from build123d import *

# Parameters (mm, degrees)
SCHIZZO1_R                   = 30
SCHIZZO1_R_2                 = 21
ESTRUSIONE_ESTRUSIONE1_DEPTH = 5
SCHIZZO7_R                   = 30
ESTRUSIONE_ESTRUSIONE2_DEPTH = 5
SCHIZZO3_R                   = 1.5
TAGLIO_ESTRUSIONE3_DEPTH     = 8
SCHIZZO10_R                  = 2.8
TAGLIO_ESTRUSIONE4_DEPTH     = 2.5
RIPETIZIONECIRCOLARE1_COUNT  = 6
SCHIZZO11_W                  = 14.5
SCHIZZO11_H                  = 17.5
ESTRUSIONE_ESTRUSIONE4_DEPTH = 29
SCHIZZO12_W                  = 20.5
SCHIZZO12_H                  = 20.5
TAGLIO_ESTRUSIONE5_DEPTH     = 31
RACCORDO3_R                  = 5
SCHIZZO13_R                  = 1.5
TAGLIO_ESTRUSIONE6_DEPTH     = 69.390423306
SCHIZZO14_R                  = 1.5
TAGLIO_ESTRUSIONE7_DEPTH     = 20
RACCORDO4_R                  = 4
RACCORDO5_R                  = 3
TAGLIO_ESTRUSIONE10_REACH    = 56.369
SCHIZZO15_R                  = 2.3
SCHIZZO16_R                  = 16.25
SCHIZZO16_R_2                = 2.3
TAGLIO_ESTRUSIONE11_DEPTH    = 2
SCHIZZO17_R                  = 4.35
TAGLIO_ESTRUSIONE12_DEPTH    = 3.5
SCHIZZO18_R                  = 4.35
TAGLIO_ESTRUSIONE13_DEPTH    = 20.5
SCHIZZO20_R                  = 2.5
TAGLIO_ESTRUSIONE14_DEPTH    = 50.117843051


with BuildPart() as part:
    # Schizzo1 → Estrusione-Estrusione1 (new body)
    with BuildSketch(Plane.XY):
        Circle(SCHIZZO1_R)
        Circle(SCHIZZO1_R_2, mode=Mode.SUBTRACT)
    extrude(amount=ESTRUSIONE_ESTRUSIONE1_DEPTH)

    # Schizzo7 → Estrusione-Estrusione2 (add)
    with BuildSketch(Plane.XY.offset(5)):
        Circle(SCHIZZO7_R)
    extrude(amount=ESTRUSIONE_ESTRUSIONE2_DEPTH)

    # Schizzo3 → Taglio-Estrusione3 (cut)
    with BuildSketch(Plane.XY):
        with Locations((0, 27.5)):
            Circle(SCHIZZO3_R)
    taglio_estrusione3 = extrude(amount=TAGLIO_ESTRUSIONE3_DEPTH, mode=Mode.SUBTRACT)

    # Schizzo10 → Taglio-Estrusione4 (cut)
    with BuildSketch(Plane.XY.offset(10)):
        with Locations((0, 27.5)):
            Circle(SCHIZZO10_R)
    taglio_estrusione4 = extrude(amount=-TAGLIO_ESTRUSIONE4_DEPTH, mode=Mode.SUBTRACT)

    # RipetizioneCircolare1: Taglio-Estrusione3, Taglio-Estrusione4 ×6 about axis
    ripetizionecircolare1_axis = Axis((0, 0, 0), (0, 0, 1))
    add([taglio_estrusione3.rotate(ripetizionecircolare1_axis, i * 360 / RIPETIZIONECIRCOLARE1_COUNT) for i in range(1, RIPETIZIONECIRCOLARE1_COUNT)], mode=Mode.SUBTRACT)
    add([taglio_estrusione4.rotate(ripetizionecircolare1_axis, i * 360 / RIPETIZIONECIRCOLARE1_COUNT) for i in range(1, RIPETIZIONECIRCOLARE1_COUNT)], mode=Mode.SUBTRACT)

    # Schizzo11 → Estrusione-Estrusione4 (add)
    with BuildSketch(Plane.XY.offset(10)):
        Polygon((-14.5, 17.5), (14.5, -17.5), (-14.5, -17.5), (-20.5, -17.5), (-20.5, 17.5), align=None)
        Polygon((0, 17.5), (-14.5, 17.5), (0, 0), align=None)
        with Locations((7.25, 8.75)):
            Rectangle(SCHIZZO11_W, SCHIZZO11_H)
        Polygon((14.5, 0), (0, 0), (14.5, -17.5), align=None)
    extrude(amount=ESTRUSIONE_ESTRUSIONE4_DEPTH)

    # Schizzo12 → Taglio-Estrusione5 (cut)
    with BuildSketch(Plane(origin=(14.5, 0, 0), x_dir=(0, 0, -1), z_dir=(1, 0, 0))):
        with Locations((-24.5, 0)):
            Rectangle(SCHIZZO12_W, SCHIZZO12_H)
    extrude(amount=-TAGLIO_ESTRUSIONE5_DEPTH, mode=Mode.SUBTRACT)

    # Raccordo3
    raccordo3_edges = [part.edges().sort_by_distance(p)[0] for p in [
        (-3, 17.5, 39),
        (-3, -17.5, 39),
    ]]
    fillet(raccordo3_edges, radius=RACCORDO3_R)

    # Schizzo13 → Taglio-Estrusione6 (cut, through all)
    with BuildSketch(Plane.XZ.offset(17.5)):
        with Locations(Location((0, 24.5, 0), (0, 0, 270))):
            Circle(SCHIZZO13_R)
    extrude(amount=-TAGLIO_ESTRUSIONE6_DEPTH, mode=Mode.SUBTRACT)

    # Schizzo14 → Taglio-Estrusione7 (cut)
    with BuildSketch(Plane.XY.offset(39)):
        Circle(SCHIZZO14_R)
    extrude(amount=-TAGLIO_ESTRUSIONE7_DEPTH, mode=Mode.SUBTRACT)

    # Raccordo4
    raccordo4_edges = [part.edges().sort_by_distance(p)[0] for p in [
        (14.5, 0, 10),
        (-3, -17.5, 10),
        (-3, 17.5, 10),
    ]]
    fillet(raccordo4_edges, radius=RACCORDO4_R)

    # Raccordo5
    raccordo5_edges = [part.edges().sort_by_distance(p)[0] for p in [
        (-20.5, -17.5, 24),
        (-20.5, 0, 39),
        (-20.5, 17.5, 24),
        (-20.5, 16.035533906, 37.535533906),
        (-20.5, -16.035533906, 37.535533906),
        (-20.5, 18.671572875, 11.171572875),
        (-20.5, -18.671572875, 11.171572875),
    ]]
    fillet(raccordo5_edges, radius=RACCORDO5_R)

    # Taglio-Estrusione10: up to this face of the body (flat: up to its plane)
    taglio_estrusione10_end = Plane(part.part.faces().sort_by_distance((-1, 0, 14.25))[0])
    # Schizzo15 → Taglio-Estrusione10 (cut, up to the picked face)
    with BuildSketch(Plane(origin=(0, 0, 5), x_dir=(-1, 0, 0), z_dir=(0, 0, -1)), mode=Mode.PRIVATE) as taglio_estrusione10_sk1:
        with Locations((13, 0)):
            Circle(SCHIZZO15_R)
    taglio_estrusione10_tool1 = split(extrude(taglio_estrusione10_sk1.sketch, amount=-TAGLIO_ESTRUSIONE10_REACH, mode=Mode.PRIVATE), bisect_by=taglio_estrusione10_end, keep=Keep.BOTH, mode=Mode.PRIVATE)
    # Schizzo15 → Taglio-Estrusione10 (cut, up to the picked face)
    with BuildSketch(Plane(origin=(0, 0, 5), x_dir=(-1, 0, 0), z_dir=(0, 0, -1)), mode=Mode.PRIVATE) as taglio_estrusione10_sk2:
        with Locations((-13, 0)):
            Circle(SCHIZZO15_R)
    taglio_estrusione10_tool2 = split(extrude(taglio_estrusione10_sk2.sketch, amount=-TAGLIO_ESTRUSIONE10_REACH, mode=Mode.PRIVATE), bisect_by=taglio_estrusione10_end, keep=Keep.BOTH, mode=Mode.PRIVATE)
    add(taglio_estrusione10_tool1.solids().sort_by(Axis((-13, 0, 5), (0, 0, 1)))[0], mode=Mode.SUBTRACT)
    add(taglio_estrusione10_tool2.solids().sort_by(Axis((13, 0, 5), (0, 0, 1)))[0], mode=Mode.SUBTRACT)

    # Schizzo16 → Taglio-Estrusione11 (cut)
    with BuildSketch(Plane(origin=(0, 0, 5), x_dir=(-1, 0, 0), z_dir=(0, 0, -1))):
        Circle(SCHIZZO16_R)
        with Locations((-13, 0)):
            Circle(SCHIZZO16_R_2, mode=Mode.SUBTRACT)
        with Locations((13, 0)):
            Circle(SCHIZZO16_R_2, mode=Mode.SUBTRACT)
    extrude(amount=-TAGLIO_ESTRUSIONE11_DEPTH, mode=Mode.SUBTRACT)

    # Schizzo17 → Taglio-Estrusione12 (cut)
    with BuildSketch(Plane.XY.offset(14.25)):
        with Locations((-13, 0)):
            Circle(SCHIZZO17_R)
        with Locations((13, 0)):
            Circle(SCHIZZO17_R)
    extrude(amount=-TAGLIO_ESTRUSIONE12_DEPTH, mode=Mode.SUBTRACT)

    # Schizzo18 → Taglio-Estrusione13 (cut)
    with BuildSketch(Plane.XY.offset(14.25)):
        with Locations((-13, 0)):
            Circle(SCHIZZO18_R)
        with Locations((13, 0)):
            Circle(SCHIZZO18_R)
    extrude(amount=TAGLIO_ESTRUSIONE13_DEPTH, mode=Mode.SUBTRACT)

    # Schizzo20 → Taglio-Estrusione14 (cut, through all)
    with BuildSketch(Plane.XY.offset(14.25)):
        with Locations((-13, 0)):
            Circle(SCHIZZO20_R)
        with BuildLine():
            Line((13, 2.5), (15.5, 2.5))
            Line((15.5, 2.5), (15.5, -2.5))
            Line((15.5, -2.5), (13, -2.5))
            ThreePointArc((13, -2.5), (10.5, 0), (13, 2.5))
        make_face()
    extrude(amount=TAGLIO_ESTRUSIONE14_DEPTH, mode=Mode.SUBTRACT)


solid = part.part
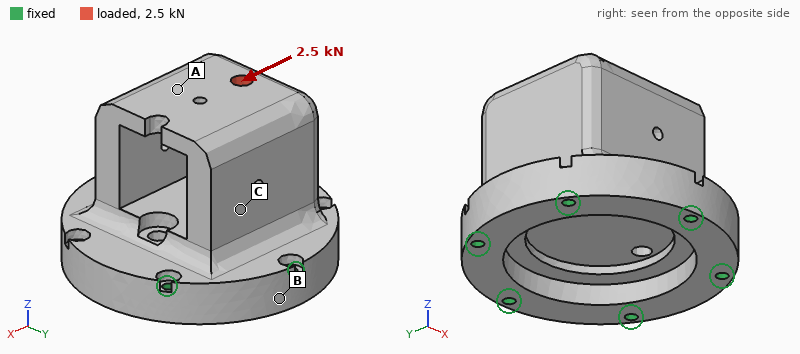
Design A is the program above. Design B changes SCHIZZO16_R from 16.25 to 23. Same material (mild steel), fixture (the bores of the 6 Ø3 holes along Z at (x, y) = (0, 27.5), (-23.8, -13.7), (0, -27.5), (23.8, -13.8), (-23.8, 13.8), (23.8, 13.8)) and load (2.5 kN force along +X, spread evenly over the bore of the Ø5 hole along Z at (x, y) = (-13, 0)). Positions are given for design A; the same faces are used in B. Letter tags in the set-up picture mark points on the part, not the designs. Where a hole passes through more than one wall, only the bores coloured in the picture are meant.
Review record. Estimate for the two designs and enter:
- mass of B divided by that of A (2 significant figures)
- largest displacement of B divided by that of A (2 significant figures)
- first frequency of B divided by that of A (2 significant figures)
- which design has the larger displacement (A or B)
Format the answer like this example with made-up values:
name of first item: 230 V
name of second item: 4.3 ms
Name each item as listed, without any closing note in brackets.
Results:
mass of B divided by that of A: 0.96
largest displacement of B divided by that of A: 1.1
first frequency of B divided by that of A: 0.97
which design has the larger displacement: B
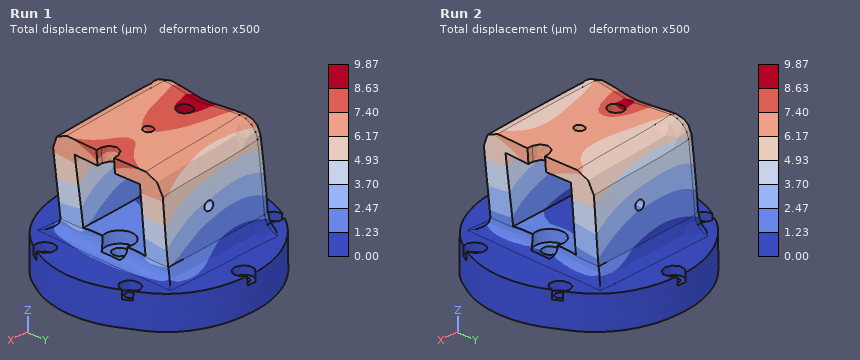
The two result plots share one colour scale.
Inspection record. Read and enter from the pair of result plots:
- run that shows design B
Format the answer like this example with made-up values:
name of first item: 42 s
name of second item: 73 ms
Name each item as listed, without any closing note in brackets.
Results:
run that shows design B: Run 1
